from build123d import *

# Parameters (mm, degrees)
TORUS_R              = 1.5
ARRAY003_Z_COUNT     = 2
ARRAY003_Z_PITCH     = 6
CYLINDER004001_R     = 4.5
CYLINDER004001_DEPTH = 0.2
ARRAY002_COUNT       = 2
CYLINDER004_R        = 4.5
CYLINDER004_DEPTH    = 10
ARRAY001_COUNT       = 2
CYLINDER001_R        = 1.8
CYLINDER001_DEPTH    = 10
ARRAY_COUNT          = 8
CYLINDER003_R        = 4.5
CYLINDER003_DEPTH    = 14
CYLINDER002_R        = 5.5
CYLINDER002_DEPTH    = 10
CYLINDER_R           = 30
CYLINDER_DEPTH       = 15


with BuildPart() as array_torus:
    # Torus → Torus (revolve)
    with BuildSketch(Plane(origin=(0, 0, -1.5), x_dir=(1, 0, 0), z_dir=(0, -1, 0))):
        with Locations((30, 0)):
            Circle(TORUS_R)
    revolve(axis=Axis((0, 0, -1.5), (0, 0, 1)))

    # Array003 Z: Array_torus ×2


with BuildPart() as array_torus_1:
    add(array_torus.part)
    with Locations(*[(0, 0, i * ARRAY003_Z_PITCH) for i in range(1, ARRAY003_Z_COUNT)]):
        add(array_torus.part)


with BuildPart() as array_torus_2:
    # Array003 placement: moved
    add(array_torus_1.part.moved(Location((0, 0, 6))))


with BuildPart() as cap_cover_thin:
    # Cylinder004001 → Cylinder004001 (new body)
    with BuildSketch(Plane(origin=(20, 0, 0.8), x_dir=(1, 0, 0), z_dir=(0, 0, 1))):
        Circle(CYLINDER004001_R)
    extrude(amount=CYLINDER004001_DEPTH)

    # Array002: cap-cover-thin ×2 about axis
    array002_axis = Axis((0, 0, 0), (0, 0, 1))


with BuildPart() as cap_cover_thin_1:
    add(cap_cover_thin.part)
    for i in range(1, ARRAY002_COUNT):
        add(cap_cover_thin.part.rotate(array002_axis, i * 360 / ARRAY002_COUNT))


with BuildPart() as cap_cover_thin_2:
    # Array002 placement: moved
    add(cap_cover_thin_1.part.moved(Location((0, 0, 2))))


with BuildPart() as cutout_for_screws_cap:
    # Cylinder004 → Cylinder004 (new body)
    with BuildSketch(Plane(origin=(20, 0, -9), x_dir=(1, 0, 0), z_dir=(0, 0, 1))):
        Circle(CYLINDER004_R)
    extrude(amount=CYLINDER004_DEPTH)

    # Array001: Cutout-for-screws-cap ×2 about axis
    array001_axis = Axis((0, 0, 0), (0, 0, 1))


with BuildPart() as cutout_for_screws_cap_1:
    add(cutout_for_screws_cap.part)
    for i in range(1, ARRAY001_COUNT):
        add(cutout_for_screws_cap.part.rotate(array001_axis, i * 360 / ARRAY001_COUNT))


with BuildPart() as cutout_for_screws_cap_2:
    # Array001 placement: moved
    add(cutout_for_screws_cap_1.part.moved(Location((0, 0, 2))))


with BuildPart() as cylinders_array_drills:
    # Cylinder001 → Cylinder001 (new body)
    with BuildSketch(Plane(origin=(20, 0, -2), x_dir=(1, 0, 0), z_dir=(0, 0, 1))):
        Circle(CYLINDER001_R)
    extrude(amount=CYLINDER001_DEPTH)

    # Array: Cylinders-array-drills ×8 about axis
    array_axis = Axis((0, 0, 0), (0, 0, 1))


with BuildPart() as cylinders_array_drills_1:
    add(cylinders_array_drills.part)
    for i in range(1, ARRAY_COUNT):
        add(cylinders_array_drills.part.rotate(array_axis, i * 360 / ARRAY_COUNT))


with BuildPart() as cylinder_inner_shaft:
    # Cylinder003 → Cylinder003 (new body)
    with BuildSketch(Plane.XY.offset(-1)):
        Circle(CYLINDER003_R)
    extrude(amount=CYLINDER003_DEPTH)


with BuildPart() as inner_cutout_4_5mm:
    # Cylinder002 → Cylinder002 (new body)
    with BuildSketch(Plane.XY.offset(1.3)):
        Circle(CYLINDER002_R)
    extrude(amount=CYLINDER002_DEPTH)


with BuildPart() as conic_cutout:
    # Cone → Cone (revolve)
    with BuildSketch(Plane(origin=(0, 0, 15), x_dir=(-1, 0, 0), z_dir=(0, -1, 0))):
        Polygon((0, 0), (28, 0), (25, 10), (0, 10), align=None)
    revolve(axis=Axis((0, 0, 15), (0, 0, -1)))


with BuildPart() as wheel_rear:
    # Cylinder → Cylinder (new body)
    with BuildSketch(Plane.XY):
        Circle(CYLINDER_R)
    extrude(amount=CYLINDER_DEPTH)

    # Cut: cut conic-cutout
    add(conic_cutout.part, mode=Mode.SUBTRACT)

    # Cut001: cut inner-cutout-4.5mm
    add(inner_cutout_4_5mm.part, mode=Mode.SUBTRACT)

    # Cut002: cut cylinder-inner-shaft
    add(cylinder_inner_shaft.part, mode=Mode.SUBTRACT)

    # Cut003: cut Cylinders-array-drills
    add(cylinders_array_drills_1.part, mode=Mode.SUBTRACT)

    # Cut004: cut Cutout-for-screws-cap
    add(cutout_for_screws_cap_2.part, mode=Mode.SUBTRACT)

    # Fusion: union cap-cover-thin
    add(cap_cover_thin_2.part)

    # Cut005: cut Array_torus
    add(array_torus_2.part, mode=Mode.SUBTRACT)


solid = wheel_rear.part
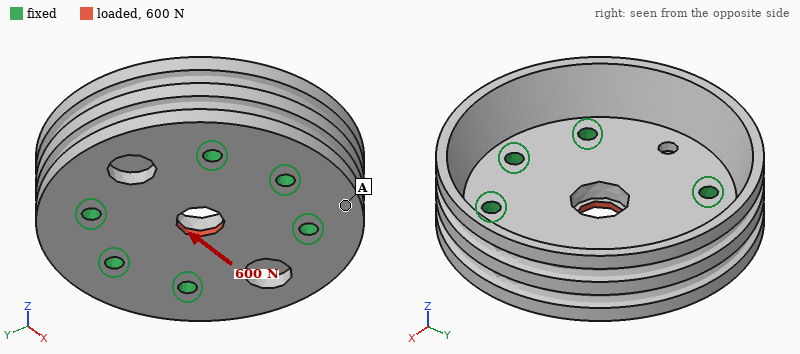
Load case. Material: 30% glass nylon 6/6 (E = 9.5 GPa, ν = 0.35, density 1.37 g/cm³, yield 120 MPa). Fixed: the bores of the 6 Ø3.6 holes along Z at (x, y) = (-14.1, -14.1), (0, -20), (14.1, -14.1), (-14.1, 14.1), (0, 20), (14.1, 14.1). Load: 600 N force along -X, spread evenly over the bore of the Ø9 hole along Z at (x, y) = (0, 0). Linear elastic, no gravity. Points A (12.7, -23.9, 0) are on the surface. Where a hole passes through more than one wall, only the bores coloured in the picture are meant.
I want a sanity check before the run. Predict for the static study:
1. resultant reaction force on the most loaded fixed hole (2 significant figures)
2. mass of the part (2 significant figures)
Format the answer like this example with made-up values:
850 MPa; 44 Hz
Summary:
140 N; 25 g
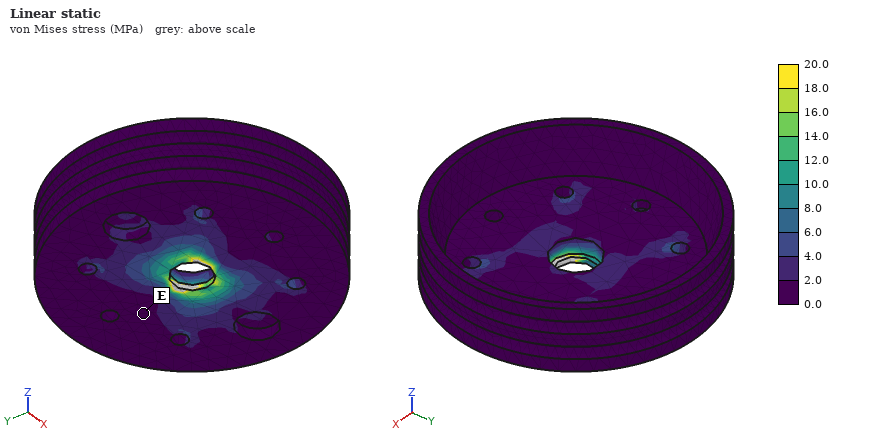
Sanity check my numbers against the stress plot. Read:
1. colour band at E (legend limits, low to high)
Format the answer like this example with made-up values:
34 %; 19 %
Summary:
0.0 to 2.0 MPa
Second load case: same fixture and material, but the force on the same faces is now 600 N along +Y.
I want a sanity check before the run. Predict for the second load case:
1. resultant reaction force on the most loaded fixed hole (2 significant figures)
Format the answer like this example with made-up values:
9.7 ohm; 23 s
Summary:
130 N
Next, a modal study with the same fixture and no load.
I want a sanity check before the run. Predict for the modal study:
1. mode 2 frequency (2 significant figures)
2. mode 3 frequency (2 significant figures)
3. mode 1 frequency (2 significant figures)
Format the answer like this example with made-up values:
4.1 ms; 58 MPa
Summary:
7000 Hz; 8900 Hz; 6500 Hz
